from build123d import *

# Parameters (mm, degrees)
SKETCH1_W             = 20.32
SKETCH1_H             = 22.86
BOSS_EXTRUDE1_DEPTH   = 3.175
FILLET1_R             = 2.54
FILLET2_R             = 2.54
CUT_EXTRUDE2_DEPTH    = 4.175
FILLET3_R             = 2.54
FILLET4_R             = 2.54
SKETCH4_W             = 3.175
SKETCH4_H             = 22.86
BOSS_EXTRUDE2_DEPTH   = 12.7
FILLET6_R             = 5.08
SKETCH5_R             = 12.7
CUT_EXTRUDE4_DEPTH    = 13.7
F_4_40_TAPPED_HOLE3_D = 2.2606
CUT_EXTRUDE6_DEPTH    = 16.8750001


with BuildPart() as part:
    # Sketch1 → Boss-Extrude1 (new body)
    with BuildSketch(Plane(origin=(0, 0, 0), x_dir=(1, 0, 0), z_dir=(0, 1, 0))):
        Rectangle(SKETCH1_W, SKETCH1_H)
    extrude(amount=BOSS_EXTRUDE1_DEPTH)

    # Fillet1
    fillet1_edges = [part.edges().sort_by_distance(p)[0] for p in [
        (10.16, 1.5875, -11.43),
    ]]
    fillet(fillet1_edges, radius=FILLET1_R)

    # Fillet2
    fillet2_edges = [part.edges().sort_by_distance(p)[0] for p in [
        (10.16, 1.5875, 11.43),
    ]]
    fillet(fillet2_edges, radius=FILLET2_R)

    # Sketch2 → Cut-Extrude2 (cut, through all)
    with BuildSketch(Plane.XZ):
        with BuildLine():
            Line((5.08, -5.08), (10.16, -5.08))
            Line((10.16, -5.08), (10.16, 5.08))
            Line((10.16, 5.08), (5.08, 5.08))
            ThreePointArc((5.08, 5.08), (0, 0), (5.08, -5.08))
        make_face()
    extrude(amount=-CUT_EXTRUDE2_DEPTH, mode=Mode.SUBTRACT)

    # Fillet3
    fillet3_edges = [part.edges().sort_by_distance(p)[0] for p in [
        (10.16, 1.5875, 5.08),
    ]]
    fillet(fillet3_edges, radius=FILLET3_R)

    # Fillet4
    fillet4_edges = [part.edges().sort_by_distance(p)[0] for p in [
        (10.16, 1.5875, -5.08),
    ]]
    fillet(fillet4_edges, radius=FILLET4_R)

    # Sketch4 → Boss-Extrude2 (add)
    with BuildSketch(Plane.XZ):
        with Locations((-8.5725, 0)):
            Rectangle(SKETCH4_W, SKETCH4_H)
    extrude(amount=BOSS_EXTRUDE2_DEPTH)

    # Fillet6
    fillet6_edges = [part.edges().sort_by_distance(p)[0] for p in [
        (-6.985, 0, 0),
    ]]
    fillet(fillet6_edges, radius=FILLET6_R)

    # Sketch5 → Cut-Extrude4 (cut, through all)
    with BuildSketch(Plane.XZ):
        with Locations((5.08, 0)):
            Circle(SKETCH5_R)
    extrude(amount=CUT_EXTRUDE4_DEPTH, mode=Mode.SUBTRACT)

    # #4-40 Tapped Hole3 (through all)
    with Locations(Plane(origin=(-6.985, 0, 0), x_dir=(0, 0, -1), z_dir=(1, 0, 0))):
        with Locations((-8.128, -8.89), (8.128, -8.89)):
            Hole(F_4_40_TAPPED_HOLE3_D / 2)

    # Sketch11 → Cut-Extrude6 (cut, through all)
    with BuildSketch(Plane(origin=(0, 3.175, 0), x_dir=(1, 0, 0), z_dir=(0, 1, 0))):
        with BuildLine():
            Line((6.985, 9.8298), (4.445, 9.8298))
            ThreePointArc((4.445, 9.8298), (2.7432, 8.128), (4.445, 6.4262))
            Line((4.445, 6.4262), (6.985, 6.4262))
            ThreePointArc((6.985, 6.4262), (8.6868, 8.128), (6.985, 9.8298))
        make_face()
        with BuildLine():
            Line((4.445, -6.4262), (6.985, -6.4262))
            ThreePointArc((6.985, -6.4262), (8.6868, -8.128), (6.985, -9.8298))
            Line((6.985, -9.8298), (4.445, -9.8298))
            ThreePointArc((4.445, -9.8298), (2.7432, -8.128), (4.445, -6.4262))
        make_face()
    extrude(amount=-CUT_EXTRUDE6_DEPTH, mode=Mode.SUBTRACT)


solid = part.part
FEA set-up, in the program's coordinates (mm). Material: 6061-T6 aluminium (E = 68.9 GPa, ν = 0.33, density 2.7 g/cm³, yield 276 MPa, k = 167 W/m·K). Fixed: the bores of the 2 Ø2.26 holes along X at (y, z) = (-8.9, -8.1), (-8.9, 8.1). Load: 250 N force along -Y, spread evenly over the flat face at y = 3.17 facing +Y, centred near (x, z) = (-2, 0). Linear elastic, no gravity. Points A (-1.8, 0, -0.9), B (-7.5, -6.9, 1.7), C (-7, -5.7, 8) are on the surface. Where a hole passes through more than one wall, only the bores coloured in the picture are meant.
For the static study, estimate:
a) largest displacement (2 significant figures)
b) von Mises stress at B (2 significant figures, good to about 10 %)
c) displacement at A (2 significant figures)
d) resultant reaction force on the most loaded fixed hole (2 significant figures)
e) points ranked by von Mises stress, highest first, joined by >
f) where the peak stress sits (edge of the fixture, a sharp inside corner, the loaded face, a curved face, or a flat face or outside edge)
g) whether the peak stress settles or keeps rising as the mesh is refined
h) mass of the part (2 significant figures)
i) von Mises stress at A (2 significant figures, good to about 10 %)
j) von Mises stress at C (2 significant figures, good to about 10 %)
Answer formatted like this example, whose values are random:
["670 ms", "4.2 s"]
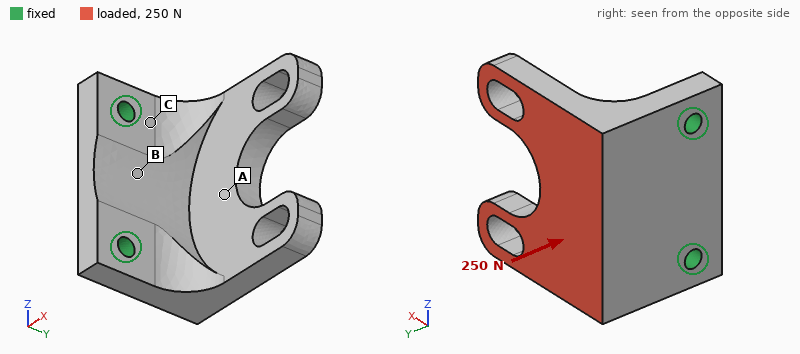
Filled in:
["89 µm", "21 MPa", "31 µm", "130 N", "C > B > A", "edge of the fixture", "keeps rising", "5.3 g", "6.3 MPa", "62 MPa"]
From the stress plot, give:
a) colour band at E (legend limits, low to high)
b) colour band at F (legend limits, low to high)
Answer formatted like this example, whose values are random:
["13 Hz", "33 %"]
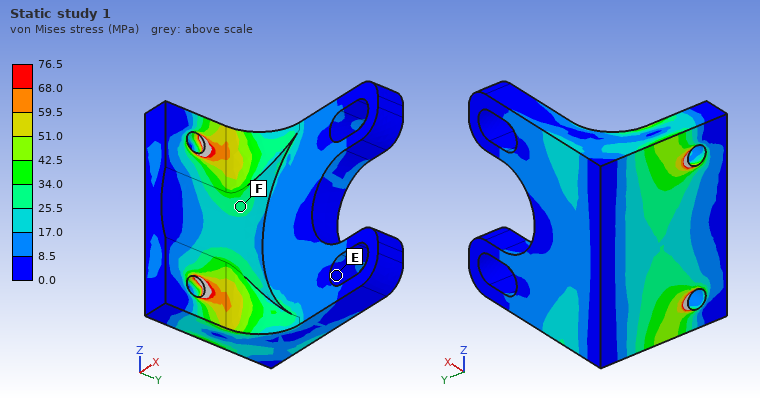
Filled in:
["0.0 to 8.5 MPa", "25.5 to 34.0 MPa"]
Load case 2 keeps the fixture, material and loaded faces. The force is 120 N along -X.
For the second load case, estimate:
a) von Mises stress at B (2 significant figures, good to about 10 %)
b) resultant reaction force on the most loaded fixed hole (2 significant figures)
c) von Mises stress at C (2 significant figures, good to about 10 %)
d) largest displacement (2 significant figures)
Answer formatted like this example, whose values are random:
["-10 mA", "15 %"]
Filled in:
["14 MPa", "60 N", "38 MPa", "48 µm"]
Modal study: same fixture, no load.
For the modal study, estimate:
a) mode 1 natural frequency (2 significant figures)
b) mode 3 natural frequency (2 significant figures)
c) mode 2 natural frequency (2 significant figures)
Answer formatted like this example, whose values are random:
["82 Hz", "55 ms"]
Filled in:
["5600 Hz", "15 kHz", "9700 Hz"]
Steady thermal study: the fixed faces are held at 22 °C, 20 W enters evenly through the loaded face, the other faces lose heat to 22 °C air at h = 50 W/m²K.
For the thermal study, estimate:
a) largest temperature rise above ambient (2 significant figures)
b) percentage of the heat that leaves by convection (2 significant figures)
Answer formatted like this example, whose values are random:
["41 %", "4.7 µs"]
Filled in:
["28 K", "4.9 %"]
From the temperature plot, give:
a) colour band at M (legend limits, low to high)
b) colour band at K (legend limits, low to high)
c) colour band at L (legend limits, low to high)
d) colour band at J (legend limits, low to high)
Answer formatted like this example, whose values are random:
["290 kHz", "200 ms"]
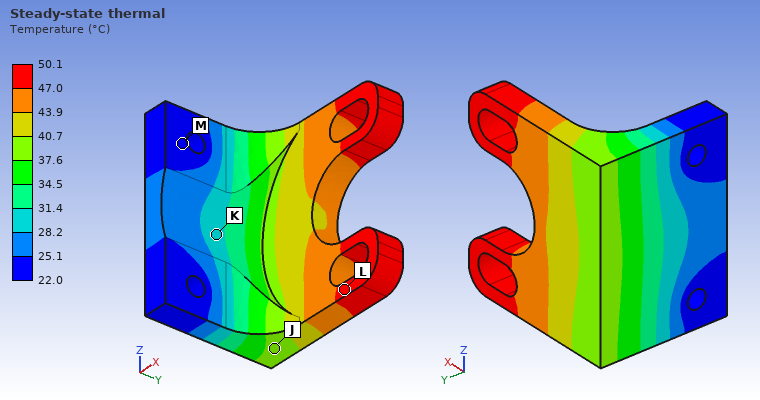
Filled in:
["22.0 to 25.1 °C", "28.2 to 31.4 °C", "47.0 to 50.1 °C", "37.6 to 40.7 °C"]
